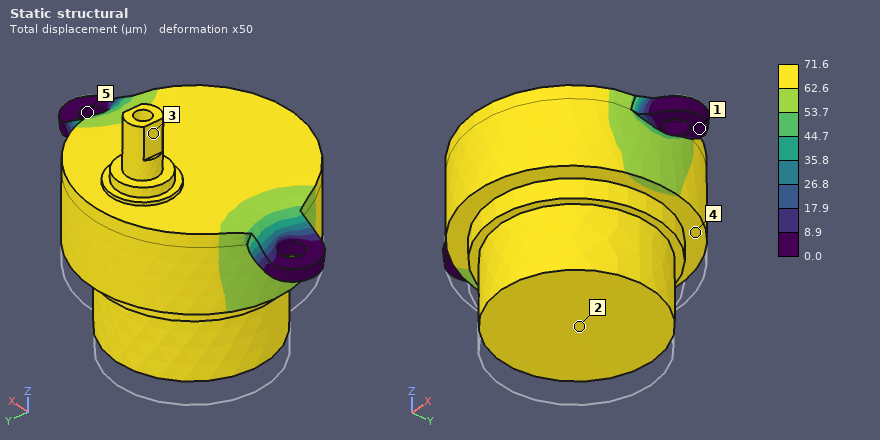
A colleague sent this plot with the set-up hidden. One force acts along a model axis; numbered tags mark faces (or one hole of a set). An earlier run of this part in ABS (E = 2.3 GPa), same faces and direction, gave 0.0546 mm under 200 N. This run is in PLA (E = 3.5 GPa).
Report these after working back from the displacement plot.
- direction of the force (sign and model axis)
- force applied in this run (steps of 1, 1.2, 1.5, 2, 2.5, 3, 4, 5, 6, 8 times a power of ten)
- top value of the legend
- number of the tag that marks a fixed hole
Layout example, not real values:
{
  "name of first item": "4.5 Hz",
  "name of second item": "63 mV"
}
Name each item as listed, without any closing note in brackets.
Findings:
{
  "direction of the force": "+Z",
  "force applied in this run": "400 N",
  "top value of the legend": "71.6 µm",
  "number of the tag that marks a fixed hole": "5"
}
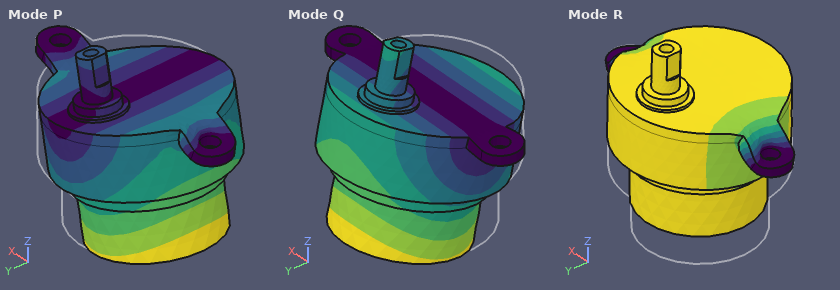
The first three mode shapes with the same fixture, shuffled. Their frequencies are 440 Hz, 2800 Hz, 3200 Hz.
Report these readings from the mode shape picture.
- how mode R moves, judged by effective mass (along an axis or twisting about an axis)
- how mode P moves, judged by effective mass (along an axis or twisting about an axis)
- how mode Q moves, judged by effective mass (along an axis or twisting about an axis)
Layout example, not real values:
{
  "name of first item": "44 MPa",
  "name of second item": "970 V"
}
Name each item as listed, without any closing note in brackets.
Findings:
{
  "how mode R moves, judged by effective mass": "along Z",
  "how mode P moves, judged by effective mass": "along X",
  "how mode Q moves, judged by effective mass": "along Y"
}
